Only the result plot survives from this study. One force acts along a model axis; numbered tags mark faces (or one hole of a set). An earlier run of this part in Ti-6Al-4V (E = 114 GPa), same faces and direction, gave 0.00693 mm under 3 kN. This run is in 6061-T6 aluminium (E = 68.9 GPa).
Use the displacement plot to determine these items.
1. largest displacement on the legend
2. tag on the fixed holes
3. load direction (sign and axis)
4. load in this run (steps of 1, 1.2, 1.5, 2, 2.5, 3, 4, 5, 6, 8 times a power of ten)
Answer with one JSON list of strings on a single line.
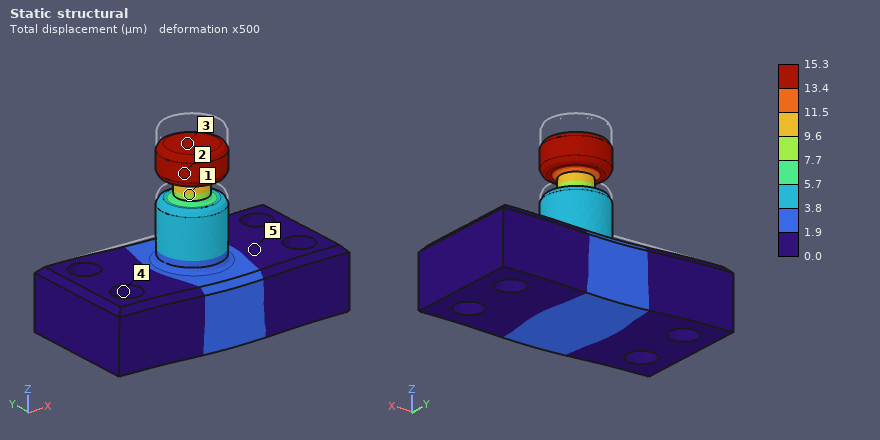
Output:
["15.3 µm", "4", "-Z", "4 kN"]
